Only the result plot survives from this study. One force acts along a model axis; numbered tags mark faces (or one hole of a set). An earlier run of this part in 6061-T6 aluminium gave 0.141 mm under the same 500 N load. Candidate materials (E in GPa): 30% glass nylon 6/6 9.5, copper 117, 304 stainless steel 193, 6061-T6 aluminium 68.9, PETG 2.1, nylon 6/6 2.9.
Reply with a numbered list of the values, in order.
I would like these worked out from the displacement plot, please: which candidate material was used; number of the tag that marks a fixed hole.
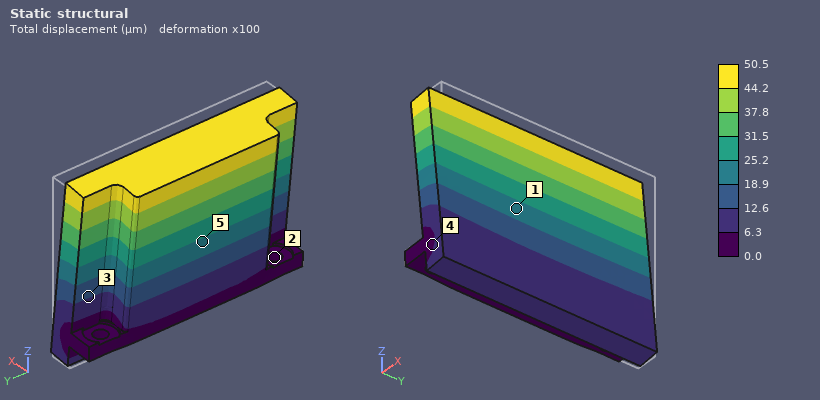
1. 304 stainless steel
2. 2
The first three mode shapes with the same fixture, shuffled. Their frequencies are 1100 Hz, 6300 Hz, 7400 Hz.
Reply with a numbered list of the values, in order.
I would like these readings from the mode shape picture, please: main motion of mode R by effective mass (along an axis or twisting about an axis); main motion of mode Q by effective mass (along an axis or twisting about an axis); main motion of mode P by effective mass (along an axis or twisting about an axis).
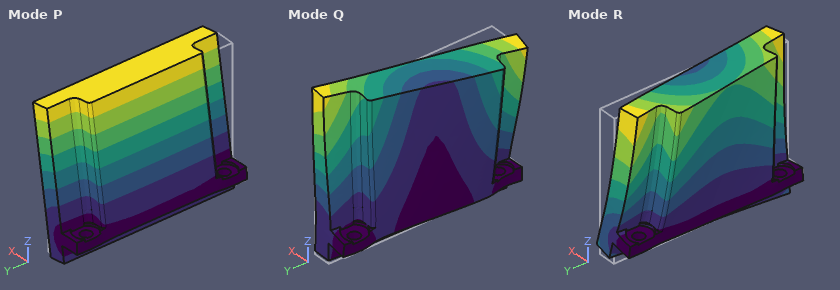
1. along Y
2. along Y
3. along X
